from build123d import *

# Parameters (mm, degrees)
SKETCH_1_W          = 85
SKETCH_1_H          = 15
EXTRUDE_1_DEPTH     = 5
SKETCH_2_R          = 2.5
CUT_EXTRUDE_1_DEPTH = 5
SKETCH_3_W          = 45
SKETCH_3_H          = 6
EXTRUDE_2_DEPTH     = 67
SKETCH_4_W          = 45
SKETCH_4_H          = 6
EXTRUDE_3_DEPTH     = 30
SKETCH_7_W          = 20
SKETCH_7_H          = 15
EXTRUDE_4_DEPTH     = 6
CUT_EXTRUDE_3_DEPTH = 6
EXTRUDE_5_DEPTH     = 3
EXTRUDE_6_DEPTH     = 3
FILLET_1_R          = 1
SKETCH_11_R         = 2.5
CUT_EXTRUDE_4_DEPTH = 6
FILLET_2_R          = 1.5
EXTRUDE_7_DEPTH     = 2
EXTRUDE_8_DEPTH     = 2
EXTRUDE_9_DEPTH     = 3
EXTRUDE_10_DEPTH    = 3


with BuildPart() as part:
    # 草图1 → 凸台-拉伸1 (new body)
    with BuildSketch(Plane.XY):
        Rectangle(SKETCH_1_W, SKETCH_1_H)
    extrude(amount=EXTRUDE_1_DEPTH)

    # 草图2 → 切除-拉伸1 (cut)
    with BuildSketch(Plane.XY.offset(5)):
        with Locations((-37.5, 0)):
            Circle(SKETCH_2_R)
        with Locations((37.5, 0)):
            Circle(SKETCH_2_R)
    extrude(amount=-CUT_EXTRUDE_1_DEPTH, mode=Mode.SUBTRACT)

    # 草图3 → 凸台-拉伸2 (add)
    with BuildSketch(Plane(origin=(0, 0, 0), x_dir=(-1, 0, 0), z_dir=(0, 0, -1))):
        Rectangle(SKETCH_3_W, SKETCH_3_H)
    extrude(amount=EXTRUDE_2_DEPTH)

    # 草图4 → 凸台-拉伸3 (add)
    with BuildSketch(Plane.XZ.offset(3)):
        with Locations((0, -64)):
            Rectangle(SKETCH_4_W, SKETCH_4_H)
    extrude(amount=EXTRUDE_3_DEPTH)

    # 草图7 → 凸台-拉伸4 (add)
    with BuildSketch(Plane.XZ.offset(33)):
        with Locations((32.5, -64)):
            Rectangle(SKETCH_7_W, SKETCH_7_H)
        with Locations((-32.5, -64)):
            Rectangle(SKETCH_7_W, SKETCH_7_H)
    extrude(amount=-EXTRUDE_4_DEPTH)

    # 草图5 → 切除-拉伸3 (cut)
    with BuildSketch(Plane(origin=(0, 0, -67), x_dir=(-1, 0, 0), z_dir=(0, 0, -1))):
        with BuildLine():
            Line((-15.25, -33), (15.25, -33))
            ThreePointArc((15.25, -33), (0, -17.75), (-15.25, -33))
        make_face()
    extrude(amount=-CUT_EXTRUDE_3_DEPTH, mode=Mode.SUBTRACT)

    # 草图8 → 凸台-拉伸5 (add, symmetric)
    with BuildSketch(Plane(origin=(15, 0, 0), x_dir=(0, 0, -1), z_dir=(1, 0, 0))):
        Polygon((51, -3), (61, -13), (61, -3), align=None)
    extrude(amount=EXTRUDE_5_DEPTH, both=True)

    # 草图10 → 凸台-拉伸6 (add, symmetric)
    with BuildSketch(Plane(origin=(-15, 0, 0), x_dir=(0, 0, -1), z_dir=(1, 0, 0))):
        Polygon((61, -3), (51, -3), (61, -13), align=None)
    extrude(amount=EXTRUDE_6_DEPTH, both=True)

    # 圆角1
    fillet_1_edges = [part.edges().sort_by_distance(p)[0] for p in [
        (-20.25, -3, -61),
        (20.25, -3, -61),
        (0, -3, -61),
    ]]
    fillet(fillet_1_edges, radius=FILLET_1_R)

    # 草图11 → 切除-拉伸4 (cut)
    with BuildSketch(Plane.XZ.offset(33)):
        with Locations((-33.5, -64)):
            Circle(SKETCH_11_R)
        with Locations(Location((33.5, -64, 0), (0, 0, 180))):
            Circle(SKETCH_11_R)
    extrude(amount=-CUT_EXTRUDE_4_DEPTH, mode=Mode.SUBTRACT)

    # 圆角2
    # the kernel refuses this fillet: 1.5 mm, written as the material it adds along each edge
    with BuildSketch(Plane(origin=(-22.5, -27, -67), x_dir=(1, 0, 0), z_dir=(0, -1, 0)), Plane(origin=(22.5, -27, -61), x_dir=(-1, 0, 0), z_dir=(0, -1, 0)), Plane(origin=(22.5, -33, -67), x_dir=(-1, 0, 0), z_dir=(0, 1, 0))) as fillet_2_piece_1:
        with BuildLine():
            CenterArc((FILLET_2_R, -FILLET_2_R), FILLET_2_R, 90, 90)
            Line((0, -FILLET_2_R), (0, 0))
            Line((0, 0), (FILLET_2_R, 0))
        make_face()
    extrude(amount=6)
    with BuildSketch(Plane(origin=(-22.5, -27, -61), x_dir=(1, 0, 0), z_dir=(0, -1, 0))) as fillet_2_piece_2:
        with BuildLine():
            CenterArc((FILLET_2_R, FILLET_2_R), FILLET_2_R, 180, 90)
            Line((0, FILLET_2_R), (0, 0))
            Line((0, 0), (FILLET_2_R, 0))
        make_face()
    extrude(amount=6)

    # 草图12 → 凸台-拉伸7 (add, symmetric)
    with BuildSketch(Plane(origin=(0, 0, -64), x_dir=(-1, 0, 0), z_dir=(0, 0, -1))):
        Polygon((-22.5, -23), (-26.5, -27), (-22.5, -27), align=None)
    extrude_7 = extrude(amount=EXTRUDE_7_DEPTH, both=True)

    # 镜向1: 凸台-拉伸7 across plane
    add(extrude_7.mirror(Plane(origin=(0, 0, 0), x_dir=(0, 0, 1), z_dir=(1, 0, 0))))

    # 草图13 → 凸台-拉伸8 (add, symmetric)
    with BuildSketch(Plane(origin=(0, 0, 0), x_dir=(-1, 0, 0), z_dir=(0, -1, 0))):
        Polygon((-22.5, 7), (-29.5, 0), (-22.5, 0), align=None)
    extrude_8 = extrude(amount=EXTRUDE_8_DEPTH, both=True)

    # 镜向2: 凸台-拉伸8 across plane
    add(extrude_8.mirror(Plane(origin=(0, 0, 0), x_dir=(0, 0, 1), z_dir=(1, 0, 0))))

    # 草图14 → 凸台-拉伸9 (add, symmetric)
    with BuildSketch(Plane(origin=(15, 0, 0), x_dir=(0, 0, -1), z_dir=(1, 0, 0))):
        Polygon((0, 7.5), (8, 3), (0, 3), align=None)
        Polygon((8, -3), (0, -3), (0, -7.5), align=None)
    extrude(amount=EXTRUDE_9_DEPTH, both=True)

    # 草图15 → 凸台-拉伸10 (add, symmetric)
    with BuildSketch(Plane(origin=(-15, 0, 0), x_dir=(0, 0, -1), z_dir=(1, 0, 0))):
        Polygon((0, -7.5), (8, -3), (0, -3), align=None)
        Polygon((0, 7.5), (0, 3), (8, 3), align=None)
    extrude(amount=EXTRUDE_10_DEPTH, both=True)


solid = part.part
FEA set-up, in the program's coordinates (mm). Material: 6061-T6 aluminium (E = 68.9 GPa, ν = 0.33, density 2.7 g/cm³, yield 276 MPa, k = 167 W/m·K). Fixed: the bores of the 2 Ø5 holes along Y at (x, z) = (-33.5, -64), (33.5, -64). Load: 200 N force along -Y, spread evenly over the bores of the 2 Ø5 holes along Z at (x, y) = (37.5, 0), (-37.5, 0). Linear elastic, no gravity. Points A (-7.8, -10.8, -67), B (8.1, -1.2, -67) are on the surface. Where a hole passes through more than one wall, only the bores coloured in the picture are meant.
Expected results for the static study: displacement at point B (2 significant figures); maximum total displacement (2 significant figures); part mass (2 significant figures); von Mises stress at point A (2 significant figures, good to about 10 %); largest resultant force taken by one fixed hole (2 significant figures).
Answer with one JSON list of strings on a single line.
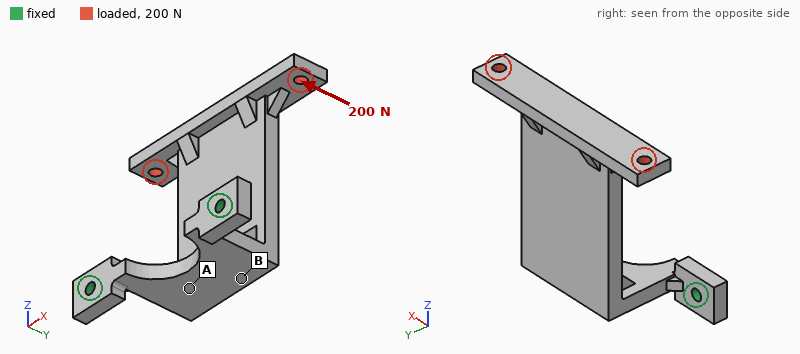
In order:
["0.30 mm", "1.3 mm", "94 g", "31 MPa", "130 N"]
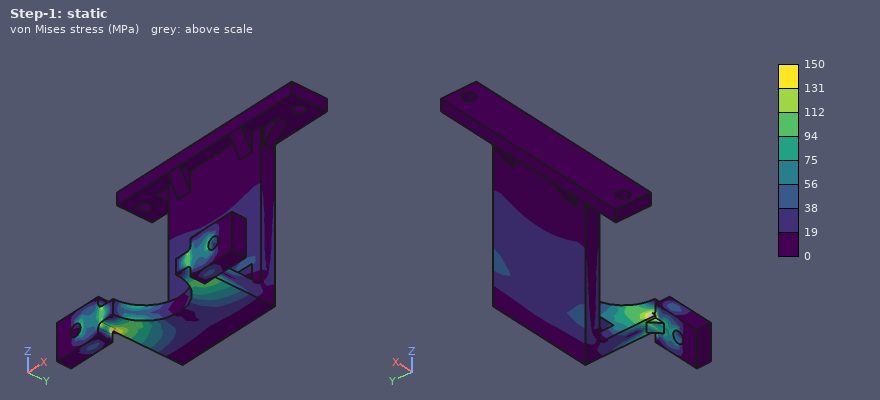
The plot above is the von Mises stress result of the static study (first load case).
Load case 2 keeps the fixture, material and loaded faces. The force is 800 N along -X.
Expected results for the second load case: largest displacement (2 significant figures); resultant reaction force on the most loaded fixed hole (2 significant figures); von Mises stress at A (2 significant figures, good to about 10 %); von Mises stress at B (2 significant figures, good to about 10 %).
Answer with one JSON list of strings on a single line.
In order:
["1.0 mm", "1.2 kN", "96 MPa", "76 MPa"]
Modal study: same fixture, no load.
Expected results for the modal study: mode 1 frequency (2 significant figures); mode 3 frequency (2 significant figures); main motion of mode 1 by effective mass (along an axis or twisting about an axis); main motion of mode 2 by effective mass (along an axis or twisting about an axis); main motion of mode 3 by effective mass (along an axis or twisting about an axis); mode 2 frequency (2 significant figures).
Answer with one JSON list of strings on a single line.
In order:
["340 Hz", "1500 Hz", "along Y", "along X", "along Z", "810 Hz"]
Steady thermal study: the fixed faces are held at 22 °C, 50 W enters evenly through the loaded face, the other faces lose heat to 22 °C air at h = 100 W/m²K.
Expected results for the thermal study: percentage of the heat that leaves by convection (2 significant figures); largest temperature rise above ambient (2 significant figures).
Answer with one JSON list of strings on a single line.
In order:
["80 %", "81 K"]
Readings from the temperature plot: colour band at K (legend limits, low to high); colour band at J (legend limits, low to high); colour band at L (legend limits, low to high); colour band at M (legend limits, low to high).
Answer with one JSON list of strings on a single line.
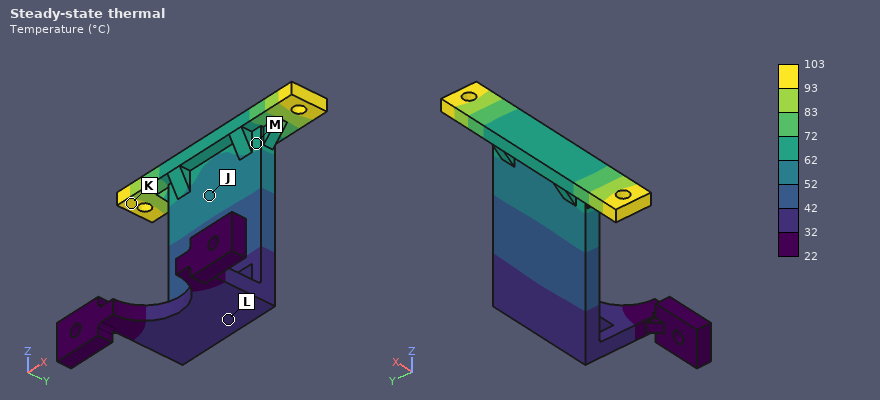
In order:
["93 to 103 °C", "52 to 62 °C", "32 to 42 °C", "62 to 72 °C"]
